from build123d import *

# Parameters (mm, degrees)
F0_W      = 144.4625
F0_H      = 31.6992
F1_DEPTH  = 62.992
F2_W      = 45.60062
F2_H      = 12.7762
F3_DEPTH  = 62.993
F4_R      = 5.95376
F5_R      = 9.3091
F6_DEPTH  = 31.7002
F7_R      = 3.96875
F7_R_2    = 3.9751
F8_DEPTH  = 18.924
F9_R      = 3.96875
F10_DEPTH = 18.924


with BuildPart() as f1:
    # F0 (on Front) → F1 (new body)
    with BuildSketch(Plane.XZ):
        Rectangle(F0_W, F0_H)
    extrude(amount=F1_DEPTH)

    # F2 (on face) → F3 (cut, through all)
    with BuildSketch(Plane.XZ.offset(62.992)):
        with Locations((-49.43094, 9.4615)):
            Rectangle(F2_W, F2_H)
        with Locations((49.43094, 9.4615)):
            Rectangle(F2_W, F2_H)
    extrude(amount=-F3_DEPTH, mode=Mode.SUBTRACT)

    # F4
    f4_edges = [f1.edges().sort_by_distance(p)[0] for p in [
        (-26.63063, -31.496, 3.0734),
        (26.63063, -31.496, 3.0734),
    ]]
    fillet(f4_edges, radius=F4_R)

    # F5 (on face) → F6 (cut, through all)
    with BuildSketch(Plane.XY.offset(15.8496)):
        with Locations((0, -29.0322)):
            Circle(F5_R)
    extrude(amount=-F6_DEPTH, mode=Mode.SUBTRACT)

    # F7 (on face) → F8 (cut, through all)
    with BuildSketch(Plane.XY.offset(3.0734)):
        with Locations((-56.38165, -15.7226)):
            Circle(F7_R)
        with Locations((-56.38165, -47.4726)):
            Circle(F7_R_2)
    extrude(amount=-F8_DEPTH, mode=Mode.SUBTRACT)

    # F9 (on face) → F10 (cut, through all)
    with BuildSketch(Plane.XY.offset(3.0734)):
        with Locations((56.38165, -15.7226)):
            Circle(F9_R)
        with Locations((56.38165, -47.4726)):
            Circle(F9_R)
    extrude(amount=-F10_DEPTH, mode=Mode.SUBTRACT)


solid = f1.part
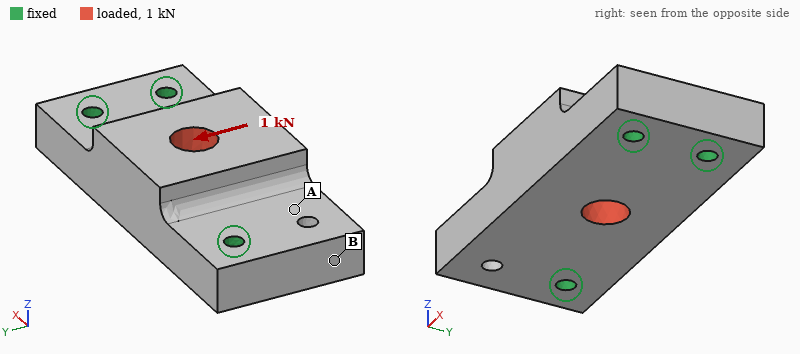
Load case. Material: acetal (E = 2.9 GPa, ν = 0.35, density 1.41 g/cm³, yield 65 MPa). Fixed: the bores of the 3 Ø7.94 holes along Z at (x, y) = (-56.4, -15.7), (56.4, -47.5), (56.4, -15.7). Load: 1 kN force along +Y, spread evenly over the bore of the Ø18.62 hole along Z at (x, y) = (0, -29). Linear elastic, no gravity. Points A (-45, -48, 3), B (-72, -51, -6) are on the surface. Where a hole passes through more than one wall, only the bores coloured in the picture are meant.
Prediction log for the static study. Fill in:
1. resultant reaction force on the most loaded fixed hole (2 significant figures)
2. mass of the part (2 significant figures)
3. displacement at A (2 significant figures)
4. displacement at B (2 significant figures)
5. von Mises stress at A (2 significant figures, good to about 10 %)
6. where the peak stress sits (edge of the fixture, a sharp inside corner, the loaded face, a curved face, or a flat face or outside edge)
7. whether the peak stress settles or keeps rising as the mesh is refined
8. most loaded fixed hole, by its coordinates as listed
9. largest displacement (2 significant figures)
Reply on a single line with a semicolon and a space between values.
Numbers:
500 N; 290 g; 24 µm; 15 µm; 0.85 MPa; edge of the fixture; keeps rising; (56.4, -15.7); 57 µm
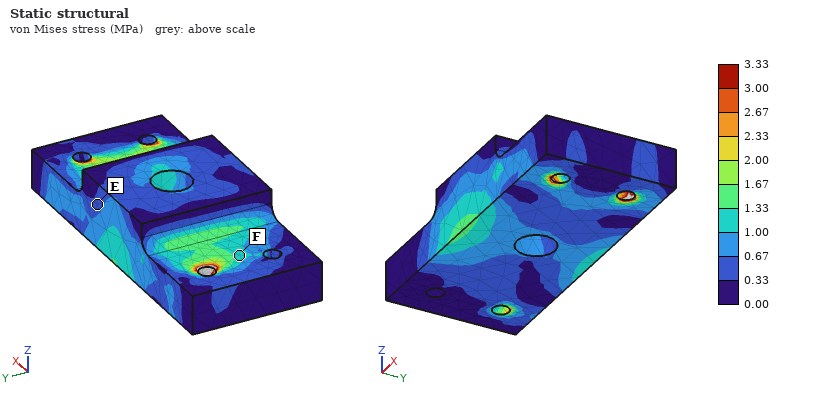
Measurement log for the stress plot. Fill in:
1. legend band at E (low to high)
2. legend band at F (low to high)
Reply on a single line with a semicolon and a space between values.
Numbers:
0.33 to 0.67 MPa; 1.00 to 1.33 MPa
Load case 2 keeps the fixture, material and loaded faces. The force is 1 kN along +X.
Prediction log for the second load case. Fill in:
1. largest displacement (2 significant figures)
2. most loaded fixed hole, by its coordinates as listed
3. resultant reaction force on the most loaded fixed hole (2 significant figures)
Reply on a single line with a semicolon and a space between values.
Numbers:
16 µm; (-56.4, -15.7); 390 N
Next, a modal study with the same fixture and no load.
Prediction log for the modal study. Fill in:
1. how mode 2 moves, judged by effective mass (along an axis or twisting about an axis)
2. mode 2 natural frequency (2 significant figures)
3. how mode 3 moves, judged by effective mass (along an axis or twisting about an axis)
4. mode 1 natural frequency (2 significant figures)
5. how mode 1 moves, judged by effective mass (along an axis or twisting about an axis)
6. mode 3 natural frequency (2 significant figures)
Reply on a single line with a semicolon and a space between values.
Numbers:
along Z; 1900 Hz; along Y; 1300 Hz; along Z; 2400 Hz
